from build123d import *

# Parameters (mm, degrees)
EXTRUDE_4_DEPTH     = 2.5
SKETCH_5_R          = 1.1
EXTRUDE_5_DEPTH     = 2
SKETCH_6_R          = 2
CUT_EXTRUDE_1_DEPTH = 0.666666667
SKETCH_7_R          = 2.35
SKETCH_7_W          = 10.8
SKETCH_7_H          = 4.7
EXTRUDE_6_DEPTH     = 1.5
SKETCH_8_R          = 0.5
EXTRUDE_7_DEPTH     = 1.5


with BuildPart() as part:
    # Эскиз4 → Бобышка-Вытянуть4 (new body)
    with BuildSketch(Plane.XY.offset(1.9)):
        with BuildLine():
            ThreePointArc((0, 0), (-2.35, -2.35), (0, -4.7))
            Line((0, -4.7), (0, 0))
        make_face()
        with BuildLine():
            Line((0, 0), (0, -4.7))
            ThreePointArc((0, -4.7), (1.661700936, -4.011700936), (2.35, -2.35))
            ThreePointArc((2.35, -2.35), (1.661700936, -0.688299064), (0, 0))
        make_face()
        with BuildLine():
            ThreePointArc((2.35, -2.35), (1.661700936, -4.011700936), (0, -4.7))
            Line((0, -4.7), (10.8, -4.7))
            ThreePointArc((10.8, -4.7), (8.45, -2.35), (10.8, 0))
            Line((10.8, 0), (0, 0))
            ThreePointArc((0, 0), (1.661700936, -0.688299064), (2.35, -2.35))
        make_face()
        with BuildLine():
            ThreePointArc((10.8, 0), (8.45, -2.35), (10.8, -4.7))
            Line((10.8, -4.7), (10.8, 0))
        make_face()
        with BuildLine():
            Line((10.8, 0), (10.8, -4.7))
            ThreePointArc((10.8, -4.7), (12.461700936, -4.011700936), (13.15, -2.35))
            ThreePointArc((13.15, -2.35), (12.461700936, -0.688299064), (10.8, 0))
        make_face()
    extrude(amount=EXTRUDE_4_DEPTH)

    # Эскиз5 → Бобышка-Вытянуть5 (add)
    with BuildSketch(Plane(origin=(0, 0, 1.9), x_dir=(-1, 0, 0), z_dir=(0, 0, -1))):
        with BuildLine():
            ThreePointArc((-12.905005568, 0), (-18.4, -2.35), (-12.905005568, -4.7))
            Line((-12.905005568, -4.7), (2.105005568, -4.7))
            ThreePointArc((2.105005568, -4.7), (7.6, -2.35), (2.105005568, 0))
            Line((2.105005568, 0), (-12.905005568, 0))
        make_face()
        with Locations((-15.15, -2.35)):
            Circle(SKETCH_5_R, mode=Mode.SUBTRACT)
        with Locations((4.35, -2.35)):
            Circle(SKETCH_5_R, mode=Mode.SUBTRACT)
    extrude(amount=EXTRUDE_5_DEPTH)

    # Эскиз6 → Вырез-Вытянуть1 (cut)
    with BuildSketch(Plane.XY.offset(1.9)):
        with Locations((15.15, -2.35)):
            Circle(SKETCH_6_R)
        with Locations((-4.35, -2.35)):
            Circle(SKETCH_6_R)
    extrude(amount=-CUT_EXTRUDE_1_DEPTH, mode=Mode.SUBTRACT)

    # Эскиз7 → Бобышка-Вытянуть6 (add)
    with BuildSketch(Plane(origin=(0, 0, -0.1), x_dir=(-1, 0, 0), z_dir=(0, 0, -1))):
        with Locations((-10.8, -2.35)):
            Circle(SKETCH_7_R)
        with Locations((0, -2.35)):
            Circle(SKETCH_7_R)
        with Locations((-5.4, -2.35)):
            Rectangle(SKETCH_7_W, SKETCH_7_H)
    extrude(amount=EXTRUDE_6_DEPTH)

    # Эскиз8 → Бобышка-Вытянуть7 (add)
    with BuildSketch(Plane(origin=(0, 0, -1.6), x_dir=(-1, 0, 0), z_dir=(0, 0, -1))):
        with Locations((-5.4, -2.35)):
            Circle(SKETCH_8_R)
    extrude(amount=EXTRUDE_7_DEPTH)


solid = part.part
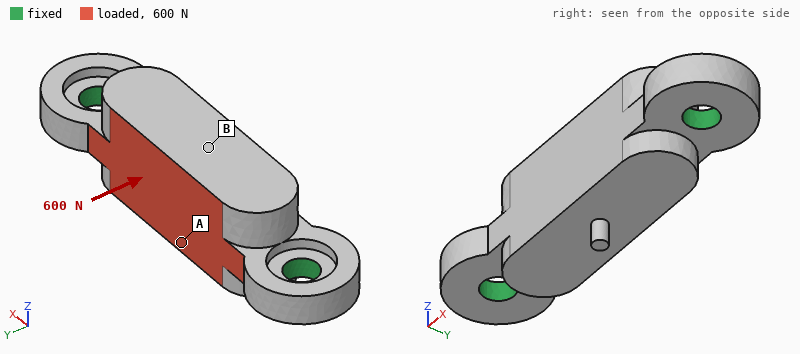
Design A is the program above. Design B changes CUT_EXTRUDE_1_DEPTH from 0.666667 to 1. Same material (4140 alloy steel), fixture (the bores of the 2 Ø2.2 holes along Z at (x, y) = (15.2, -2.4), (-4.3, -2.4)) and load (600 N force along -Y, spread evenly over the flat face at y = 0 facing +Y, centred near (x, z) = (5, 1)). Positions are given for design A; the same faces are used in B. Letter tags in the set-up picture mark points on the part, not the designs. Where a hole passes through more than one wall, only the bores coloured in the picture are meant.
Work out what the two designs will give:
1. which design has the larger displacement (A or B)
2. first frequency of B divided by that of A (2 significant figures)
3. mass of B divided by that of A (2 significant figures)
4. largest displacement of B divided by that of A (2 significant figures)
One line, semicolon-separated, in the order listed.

B; 0.86; 0.99; 1.3
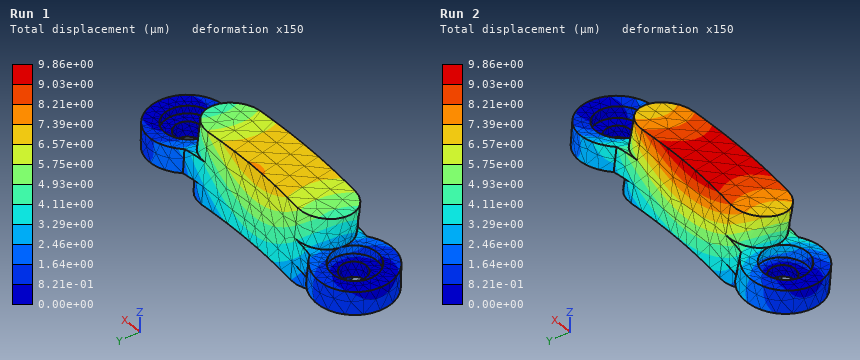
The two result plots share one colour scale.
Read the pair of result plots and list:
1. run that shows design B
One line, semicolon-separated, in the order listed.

Run 2
